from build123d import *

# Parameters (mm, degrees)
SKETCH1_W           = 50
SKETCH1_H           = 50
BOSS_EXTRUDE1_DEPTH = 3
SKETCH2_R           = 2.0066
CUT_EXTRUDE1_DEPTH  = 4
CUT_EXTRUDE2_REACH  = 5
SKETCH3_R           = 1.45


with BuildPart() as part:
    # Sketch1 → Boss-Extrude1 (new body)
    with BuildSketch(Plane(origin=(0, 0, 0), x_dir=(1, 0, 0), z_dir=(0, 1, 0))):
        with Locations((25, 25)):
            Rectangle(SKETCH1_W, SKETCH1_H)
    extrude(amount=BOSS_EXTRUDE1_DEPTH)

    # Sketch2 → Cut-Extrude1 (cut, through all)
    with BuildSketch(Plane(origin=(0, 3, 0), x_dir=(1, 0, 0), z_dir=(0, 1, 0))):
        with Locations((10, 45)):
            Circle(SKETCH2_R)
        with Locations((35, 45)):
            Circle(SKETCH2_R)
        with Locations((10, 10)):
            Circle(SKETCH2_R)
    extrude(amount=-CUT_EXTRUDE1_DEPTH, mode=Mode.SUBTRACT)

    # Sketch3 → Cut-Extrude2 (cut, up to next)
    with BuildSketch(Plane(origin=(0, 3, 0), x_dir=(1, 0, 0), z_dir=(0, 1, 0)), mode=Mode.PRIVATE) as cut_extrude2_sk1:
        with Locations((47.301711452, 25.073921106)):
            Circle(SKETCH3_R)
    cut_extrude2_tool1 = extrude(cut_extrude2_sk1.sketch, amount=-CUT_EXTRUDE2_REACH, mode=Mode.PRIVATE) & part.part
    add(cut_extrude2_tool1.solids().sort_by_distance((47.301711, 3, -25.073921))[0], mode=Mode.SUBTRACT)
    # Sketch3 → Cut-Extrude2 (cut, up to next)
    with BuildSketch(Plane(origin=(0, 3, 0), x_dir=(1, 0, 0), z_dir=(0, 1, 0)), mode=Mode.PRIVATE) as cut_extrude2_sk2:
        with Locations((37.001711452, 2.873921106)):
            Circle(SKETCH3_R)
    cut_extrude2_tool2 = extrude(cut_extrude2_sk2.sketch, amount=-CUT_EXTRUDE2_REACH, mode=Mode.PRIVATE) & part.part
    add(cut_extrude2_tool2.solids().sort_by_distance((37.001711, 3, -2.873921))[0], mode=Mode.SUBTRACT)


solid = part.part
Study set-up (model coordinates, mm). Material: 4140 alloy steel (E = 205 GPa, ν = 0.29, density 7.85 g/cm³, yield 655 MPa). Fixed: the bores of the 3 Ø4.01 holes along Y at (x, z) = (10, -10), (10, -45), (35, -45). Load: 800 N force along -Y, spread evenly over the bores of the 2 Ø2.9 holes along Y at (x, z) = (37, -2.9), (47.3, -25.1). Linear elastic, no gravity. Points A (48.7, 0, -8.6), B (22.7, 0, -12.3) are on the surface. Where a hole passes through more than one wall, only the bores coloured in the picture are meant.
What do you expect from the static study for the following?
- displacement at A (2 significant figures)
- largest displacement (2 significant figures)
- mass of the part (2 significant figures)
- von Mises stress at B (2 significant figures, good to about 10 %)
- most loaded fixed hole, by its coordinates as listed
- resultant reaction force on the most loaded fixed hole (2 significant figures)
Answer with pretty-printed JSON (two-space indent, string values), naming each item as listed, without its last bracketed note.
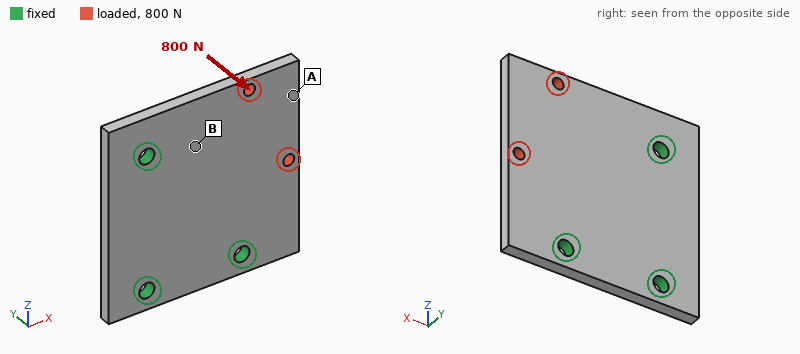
{
  "displacement at A": "0.29 mm",
  "largest displacement": "0.37 mm",
  "mass of the part": "58 g",
  "von Mises stress at B": "140 MPa",
  "most loaded fixed hole, by its coordinates as listed": "(35, -45)",
  "resultant reaction force on the most loaded fixed hole": "560 N"
}
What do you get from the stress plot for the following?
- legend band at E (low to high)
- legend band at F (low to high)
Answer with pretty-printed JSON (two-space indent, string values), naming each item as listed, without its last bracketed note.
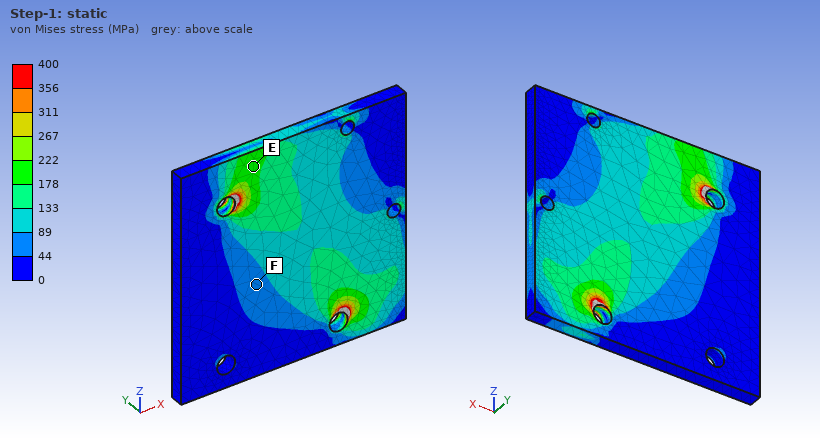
{
  "legend band at E": "178 to 222 MPa",
  "legend band at F": "44 to 89 MPa"
}
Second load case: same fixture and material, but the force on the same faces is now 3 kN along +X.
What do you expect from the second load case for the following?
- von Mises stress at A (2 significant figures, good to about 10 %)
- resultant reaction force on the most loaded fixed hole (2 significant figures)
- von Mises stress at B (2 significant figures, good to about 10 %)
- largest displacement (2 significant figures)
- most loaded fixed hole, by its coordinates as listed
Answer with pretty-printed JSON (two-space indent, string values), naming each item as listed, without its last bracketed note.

{
  "von Mises stress at A": "13 MPa",
  "resultant reaction force on the most loaded fixed hole": "2.3 kN",
  "von Mises stress at B": "35 MPa",
  "largest displacement": "8.7 µm",
  "most loaded fixed hole, by its coordinates as listed": "(10, -10)"
}
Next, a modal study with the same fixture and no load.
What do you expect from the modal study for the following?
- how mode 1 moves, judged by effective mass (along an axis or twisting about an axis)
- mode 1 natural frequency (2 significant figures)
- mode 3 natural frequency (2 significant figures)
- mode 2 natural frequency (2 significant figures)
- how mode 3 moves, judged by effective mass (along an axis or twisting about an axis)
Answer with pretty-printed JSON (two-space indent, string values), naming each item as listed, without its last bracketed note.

{
  "how mode 1 moves, judged by effective mass": "along Y",
  "mode 1 natural frequency": "2600 Hz",
  "mode 3 natural frequency": "9800 Hz",
  "mode 2 natural frequency": "7700 Hz",
  "how mode 3 moves, judged by effective mass": "along Y"
}
